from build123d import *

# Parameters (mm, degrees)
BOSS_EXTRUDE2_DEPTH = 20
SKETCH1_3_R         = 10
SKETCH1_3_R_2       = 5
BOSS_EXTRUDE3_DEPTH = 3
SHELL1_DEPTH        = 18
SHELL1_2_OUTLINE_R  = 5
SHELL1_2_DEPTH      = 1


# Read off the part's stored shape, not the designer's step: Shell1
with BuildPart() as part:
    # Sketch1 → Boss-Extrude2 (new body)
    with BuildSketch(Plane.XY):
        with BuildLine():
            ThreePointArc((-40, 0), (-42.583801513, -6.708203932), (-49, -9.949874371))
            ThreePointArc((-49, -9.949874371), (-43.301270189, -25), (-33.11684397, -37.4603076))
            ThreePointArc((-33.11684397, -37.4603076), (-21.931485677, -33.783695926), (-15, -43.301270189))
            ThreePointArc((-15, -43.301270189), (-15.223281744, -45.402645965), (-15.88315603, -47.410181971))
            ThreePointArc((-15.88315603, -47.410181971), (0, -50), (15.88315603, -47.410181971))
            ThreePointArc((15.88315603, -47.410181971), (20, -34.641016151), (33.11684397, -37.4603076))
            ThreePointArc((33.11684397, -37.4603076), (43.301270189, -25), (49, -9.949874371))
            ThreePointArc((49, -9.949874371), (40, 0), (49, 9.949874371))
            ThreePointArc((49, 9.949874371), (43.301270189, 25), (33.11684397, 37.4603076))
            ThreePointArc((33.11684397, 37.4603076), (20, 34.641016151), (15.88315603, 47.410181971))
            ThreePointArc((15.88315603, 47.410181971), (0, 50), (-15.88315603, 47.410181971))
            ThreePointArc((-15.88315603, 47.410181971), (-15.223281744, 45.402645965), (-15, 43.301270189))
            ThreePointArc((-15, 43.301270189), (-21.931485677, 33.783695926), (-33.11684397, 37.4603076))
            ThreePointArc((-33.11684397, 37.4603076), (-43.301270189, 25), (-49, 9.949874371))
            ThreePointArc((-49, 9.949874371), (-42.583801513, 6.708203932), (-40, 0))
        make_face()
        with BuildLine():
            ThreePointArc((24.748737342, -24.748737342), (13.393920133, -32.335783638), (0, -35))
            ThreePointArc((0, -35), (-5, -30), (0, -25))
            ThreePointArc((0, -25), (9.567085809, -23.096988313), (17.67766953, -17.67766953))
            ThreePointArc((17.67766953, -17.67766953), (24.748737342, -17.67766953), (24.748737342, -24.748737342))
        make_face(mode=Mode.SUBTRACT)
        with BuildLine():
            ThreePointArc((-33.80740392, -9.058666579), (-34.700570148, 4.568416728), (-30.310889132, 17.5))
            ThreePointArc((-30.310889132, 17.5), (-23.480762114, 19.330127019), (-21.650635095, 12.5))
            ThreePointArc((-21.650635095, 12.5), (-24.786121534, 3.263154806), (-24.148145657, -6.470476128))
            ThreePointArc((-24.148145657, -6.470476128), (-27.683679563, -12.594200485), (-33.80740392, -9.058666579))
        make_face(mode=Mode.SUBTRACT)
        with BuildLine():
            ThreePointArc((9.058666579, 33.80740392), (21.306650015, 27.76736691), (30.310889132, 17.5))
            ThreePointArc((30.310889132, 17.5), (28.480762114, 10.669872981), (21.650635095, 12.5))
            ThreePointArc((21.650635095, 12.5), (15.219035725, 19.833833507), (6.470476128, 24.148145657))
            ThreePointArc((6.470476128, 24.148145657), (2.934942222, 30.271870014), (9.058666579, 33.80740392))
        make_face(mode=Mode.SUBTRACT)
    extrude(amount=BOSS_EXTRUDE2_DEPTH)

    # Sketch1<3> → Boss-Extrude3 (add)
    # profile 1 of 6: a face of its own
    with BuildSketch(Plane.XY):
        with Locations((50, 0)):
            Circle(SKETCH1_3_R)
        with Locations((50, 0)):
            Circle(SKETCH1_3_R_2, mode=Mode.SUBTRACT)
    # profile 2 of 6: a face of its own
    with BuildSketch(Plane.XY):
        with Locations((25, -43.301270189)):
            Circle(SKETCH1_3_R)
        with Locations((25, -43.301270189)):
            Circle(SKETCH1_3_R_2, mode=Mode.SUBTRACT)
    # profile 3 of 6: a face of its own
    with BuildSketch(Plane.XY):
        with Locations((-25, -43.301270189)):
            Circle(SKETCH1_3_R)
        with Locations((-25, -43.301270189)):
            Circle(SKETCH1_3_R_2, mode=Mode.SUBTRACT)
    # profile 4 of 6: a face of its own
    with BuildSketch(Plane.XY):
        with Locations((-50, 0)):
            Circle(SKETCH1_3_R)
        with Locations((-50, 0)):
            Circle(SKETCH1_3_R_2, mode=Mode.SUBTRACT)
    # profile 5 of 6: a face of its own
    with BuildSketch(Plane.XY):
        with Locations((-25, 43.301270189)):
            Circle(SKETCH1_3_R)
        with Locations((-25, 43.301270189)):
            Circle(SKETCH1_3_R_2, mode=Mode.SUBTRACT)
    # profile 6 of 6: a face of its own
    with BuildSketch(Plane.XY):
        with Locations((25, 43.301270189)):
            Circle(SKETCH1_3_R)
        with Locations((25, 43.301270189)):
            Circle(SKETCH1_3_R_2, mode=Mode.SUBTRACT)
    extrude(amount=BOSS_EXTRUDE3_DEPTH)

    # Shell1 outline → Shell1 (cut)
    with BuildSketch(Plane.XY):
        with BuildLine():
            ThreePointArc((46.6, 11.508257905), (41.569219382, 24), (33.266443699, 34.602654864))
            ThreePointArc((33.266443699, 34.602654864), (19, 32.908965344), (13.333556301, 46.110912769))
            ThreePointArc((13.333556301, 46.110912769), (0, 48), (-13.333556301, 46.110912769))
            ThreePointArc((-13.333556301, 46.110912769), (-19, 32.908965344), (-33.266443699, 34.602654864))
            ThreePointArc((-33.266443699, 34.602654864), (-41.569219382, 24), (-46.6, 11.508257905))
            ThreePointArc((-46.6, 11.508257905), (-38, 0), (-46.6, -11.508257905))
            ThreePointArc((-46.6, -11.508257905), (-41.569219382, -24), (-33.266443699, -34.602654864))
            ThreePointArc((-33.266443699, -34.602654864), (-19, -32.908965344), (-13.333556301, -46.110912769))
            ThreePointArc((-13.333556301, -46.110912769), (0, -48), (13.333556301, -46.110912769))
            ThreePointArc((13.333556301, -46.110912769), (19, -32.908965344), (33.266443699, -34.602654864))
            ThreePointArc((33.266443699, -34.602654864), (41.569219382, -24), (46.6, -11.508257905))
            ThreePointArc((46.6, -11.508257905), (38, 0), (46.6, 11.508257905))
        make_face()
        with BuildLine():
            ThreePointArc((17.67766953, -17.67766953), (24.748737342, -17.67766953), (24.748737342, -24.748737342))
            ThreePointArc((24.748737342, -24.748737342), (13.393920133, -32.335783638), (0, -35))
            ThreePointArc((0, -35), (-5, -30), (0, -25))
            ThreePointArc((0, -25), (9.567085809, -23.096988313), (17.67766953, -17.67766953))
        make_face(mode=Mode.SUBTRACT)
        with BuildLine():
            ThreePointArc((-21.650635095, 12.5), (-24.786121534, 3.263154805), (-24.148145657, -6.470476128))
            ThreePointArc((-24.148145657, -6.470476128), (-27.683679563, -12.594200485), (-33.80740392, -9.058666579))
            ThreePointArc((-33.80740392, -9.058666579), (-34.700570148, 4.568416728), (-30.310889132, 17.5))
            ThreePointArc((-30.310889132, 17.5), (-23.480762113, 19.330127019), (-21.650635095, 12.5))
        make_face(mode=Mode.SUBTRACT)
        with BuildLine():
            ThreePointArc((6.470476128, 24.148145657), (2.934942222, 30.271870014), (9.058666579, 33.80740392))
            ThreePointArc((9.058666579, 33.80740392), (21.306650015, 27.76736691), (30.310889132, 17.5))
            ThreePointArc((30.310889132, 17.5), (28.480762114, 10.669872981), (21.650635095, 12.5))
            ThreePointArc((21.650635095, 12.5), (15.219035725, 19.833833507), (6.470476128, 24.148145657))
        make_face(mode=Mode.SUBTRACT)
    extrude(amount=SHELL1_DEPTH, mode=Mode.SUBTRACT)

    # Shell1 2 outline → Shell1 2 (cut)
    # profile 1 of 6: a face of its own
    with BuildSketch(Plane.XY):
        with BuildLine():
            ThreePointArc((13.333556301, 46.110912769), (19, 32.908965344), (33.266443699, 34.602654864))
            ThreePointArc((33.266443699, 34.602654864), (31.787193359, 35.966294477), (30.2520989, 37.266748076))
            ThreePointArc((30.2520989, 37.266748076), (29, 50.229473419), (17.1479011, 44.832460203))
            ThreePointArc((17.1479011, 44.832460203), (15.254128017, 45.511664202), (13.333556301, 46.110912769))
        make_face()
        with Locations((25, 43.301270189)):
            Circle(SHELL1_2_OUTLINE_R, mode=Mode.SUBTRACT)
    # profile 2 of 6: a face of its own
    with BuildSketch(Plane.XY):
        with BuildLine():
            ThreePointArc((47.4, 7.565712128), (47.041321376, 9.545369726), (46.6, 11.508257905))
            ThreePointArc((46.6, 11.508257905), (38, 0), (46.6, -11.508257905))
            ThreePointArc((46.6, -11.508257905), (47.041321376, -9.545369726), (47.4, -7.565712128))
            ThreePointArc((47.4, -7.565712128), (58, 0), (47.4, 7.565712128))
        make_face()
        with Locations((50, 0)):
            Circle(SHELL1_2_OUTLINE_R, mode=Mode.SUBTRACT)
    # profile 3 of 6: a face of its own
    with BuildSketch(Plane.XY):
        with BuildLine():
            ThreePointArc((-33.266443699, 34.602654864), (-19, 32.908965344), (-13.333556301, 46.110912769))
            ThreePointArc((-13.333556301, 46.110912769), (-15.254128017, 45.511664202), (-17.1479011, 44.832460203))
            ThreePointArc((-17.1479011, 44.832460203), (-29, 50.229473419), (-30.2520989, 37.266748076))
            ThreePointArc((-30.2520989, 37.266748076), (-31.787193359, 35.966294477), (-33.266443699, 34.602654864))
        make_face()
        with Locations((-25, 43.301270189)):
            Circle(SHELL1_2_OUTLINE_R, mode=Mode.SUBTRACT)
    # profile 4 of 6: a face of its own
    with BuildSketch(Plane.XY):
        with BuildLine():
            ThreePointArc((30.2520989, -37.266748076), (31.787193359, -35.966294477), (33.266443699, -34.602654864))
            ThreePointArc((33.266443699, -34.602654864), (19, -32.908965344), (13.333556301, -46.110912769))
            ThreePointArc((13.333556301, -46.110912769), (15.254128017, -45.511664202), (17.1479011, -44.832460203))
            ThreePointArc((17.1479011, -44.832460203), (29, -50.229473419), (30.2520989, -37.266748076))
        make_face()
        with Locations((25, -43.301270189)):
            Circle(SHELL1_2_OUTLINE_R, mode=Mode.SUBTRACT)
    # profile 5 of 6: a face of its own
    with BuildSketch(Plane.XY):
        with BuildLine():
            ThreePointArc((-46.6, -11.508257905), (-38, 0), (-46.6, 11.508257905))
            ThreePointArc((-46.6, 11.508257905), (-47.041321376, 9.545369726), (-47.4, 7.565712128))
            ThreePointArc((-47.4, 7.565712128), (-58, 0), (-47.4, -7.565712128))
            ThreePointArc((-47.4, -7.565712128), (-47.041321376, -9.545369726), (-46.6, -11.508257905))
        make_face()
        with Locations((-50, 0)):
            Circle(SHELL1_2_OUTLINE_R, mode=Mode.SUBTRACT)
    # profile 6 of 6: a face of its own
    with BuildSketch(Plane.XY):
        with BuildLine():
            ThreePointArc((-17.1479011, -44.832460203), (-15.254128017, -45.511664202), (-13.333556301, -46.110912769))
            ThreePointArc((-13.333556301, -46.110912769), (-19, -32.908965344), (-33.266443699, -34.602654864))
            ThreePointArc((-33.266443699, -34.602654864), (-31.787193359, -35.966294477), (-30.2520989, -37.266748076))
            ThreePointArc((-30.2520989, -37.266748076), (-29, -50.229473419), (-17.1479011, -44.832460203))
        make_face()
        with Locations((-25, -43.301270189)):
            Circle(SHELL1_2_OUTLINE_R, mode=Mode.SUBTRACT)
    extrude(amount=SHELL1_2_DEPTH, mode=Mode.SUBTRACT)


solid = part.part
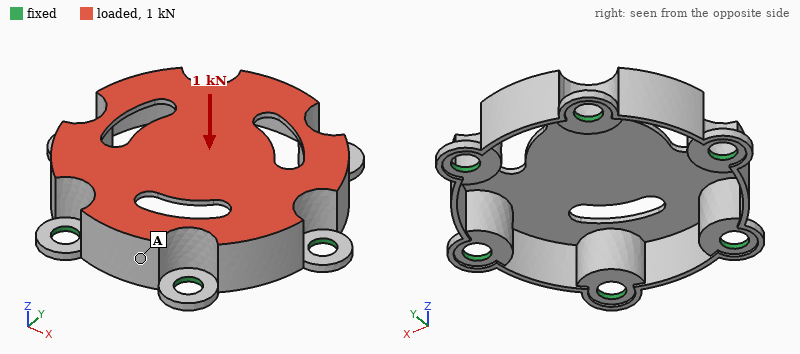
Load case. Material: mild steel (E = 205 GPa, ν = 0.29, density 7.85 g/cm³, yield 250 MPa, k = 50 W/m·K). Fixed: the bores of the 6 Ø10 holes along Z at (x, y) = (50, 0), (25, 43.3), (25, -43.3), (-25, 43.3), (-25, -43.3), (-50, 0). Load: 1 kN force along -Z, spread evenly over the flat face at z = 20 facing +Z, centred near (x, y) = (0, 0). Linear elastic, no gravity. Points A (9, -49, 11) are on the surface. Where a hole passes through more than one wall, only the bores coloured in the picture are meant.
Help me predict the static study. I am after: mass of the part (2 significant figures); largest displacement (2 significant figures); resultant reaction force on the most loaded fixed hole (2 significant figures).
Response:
220 g
77 µm
230 N
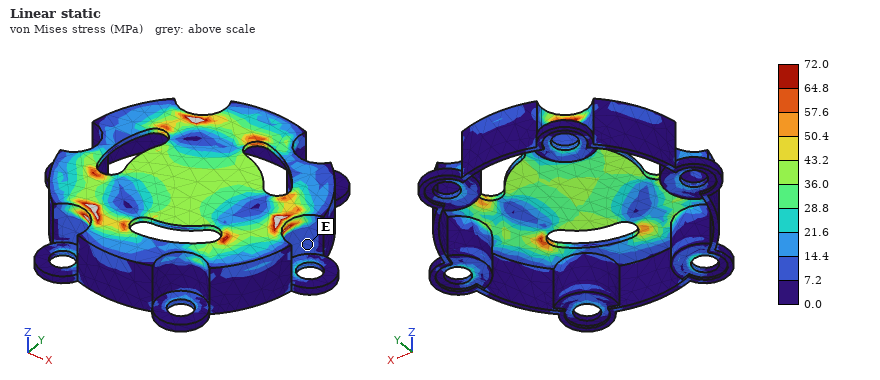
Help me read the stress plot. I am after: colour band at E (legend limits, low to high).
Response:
7.2 to 14.4 MPa
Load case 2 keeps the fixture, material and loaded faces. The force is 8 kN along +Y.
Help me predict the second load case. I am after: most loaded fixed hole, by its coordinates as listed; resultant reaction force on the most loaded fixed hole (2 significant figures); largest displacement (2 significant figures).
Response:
(50, 0)
2.5 kN
45 µm
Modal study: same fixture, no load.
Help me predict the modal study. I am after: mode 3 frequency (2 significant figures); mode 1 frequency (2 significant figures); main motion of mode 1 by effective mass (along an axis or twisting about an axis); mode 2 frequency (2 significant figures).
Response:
4300 Hz
2200 Hz
along Z
4300 Hz
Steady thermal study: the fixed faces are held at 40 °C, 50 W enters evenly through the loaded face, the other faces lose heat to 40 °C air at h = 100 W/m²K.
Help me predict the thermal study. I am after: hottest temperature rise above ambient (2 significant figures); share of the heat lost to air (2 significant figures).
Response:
46 K
68 %
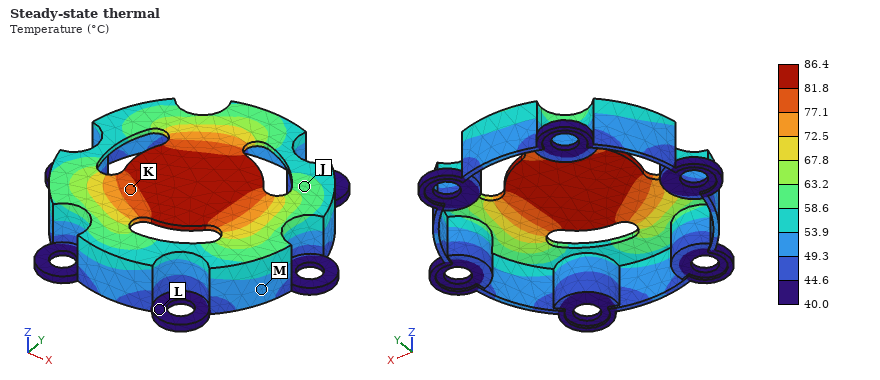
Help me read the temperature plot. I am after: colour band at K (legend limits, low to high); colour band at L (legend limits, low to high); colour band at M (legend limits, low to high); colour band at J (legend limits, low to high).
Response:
77.1 to 81.8 °C
40.0 to 44.6 °C
49.3 to 53.9 °C
58.6 to 63.2 °C
